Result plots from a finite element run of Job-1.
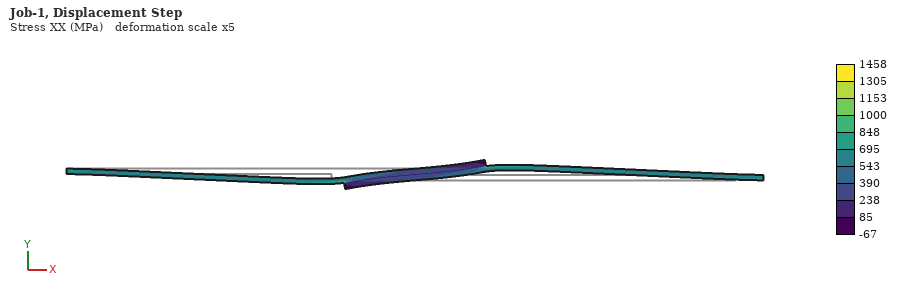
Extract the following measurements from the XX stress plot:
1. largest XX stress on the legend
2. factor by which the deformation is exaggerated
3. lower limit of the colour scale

1458 MPa
5
-67 MPa
